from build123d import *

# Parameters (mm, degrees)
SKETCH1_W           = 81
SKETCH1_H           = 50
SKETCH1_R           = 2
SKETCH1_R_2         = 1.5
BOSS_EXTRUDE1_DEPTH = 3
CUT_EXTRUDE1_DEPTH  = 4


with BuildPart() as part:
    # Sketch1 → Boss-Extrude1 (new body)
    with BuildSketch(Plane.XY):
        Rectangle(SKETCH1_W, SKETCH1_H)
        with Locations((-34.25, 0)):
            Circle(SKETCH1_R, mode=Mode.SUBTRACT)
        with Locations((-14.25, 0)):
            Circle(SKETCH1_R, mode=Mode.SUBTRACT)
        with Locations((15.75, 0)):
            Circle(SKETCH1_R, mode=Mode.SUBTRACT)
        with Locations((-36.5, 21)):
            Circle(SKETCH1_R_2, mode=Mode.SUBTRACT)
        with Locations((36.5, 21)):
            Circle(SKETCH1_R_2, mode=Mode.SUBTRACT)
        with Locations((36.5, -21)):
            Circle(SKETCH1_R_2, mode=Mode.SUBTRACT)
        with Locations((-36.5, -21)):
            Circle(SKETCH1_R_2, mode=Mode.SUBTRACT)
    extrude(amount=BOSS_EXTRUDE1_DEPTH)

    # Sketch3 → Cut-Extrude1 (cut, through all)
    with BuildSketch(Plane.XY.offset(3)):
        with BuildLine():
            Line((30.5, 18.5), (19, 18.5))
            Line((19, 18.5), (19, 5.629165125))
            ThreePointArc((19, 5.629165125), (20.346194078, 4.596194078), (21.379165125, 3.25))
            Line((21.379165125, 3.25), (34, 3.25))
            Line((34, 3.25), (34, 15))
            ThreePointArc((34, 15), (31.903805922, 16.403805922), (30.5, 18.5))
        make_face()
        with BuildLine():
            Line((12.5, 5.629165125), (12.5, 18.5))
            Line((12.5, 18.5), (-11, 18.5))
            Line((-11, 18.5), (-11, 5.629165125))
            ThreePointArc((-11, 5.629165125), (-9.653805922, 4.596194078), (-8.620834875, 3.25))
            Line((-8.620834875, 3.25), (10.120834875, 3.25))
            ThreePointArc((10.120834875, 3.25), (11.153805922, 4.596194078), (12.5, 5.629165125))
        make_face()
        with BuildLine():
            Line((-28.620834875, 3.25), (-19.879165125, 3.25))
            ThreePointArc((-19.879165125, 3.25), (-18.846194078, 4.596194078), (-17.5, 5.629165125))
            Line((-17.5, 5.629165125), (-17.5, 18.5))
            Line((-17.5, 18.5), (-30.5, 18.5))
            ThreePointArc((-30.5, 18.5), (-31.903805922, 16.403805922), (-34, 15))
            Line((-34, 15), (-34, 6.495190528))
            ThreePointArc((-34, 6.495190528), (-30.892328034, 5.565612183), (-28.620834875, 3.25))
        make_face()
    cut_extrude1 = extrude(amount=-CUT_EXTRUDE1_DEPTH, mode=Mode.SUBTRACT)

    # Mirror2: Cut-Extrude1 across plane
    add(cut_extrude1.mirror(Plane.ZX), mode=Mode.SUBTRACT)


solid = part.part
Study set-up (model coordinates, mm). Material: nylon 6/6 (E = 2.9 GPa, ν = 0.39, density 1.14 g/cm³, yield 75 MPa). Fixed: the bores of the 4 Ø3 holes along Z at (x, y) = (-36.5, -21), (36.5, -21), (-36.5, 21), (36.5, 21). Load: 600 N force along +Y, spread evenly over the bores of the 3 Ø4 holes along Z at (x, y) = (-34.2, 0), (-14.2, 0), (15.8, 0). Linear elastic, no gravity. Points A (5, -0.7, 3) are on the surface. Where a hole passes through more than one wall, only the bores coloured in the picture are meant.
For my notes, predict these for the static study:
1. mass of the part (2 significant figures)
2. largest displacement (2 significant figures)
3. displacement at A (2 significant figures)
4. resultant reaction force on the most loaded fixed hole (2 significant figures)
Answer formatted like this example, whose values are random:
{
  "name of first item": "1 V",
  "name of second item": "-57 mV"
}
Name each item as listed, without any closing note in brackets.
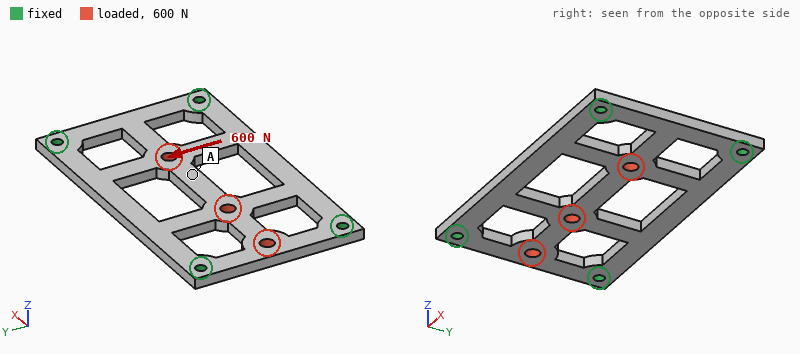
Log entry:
{
  "mass of the part": "8.2 g",
  "largest displacement": "0.34 mm",
  "displacement at A": "0.32 mm",
  "resultant reaction force on the most loaded fixed hole": "210 N"
}
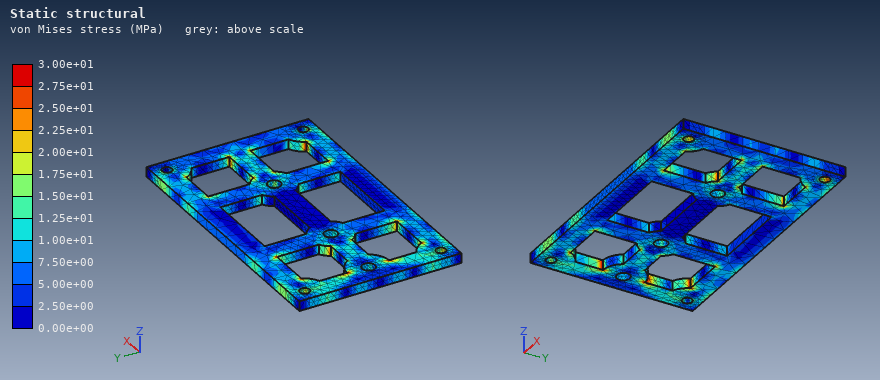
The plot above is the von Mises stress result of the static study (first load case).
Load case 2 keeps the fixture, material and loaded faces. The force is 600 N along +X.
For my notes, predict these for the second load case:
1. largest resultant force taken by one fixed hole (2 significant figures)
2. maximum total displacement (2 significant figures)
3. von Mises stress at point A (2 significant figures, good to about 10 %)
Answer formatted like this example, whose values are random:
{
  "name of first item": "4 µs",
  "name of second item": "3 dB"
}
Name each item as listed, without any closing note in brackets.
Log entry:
{
  "largest resultant force taken by one fixed hole": "170 N",
  "maximum total displacement": "0.31 mm",
  "von Mises stress at point A": "2.8 MPa"
}
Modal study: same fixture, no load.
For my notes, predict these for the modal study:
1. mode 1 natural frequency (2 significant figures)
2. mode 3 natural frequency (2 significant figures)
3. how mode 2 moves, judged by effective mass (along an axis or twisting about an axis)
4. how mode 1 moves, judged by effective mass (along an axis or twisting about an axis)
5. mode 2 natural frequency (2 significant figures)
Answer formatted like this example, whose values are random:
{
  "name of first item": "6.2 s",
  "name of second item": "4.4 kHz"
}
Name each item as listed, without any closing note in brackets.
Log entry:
{
  "mode 1 natural frequency": "770 Hz",
  "mode 3 natural frequency": "1700 Hz",
  "how mode 2 moves, judged by effective mass": "twisting about X",
  "how mode 1 moves, judged by effective mass": "along Z",
  "mode 2 natural frequency": "1100 Hz"
}
